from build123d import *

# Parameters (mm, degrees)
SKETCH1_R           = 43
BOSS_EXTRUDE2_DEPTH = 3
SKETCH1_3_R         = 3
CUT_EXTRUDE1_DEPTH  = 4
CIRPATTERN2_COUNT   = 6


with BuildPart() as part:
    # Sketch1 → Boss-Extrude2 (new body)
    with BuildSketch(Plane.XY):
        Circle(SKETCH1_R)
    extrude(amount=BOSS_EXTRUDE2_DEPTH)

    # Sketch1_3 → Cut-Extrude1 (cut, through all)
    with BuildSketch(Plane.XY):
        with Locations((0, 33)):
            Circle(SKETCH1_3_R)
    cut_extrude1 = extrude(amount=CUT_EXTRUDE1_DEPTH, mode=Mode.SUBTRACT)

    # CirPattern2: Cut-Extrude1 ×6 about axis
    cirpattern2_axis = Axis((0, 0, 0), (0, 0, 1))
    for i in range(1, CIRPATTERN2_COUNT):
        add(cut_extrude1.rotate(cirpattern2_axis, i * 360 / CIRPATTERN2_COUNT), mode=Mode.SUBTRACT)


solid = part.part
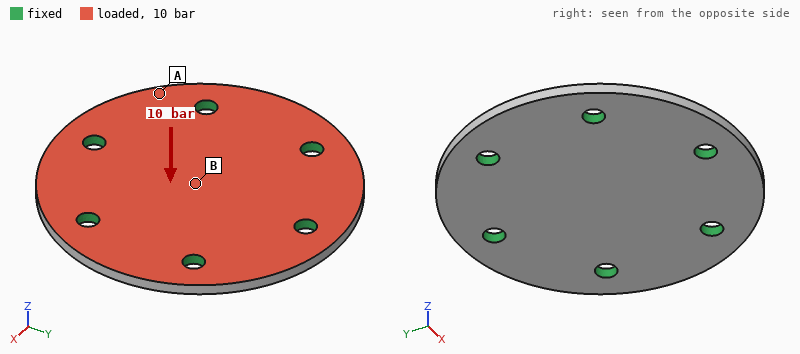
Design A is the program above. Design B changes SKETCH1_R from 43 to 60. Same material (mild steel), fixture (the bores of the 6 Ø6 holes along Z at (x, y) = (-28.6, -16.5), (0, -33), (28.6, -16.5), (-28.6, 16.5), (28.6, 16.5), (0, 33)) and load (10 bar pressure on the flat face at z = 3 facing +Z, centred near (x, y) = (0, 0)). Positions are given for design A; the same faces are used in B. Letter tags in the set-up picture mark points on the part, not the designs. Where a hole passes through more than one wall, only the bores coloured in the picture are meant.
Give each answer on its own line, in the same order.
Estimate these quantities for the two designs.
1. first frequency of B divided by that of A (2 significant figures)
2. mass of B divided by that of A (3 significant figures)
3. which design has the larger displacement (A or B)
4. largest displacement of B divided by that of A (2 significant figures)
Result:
0.47
1.98
B
4.7
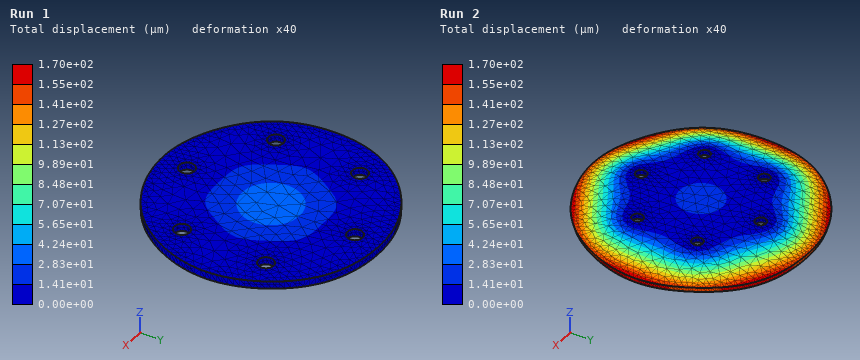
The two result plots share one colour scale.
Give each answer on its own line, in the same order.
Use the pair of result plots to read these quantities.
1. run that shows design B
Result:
Run 2
